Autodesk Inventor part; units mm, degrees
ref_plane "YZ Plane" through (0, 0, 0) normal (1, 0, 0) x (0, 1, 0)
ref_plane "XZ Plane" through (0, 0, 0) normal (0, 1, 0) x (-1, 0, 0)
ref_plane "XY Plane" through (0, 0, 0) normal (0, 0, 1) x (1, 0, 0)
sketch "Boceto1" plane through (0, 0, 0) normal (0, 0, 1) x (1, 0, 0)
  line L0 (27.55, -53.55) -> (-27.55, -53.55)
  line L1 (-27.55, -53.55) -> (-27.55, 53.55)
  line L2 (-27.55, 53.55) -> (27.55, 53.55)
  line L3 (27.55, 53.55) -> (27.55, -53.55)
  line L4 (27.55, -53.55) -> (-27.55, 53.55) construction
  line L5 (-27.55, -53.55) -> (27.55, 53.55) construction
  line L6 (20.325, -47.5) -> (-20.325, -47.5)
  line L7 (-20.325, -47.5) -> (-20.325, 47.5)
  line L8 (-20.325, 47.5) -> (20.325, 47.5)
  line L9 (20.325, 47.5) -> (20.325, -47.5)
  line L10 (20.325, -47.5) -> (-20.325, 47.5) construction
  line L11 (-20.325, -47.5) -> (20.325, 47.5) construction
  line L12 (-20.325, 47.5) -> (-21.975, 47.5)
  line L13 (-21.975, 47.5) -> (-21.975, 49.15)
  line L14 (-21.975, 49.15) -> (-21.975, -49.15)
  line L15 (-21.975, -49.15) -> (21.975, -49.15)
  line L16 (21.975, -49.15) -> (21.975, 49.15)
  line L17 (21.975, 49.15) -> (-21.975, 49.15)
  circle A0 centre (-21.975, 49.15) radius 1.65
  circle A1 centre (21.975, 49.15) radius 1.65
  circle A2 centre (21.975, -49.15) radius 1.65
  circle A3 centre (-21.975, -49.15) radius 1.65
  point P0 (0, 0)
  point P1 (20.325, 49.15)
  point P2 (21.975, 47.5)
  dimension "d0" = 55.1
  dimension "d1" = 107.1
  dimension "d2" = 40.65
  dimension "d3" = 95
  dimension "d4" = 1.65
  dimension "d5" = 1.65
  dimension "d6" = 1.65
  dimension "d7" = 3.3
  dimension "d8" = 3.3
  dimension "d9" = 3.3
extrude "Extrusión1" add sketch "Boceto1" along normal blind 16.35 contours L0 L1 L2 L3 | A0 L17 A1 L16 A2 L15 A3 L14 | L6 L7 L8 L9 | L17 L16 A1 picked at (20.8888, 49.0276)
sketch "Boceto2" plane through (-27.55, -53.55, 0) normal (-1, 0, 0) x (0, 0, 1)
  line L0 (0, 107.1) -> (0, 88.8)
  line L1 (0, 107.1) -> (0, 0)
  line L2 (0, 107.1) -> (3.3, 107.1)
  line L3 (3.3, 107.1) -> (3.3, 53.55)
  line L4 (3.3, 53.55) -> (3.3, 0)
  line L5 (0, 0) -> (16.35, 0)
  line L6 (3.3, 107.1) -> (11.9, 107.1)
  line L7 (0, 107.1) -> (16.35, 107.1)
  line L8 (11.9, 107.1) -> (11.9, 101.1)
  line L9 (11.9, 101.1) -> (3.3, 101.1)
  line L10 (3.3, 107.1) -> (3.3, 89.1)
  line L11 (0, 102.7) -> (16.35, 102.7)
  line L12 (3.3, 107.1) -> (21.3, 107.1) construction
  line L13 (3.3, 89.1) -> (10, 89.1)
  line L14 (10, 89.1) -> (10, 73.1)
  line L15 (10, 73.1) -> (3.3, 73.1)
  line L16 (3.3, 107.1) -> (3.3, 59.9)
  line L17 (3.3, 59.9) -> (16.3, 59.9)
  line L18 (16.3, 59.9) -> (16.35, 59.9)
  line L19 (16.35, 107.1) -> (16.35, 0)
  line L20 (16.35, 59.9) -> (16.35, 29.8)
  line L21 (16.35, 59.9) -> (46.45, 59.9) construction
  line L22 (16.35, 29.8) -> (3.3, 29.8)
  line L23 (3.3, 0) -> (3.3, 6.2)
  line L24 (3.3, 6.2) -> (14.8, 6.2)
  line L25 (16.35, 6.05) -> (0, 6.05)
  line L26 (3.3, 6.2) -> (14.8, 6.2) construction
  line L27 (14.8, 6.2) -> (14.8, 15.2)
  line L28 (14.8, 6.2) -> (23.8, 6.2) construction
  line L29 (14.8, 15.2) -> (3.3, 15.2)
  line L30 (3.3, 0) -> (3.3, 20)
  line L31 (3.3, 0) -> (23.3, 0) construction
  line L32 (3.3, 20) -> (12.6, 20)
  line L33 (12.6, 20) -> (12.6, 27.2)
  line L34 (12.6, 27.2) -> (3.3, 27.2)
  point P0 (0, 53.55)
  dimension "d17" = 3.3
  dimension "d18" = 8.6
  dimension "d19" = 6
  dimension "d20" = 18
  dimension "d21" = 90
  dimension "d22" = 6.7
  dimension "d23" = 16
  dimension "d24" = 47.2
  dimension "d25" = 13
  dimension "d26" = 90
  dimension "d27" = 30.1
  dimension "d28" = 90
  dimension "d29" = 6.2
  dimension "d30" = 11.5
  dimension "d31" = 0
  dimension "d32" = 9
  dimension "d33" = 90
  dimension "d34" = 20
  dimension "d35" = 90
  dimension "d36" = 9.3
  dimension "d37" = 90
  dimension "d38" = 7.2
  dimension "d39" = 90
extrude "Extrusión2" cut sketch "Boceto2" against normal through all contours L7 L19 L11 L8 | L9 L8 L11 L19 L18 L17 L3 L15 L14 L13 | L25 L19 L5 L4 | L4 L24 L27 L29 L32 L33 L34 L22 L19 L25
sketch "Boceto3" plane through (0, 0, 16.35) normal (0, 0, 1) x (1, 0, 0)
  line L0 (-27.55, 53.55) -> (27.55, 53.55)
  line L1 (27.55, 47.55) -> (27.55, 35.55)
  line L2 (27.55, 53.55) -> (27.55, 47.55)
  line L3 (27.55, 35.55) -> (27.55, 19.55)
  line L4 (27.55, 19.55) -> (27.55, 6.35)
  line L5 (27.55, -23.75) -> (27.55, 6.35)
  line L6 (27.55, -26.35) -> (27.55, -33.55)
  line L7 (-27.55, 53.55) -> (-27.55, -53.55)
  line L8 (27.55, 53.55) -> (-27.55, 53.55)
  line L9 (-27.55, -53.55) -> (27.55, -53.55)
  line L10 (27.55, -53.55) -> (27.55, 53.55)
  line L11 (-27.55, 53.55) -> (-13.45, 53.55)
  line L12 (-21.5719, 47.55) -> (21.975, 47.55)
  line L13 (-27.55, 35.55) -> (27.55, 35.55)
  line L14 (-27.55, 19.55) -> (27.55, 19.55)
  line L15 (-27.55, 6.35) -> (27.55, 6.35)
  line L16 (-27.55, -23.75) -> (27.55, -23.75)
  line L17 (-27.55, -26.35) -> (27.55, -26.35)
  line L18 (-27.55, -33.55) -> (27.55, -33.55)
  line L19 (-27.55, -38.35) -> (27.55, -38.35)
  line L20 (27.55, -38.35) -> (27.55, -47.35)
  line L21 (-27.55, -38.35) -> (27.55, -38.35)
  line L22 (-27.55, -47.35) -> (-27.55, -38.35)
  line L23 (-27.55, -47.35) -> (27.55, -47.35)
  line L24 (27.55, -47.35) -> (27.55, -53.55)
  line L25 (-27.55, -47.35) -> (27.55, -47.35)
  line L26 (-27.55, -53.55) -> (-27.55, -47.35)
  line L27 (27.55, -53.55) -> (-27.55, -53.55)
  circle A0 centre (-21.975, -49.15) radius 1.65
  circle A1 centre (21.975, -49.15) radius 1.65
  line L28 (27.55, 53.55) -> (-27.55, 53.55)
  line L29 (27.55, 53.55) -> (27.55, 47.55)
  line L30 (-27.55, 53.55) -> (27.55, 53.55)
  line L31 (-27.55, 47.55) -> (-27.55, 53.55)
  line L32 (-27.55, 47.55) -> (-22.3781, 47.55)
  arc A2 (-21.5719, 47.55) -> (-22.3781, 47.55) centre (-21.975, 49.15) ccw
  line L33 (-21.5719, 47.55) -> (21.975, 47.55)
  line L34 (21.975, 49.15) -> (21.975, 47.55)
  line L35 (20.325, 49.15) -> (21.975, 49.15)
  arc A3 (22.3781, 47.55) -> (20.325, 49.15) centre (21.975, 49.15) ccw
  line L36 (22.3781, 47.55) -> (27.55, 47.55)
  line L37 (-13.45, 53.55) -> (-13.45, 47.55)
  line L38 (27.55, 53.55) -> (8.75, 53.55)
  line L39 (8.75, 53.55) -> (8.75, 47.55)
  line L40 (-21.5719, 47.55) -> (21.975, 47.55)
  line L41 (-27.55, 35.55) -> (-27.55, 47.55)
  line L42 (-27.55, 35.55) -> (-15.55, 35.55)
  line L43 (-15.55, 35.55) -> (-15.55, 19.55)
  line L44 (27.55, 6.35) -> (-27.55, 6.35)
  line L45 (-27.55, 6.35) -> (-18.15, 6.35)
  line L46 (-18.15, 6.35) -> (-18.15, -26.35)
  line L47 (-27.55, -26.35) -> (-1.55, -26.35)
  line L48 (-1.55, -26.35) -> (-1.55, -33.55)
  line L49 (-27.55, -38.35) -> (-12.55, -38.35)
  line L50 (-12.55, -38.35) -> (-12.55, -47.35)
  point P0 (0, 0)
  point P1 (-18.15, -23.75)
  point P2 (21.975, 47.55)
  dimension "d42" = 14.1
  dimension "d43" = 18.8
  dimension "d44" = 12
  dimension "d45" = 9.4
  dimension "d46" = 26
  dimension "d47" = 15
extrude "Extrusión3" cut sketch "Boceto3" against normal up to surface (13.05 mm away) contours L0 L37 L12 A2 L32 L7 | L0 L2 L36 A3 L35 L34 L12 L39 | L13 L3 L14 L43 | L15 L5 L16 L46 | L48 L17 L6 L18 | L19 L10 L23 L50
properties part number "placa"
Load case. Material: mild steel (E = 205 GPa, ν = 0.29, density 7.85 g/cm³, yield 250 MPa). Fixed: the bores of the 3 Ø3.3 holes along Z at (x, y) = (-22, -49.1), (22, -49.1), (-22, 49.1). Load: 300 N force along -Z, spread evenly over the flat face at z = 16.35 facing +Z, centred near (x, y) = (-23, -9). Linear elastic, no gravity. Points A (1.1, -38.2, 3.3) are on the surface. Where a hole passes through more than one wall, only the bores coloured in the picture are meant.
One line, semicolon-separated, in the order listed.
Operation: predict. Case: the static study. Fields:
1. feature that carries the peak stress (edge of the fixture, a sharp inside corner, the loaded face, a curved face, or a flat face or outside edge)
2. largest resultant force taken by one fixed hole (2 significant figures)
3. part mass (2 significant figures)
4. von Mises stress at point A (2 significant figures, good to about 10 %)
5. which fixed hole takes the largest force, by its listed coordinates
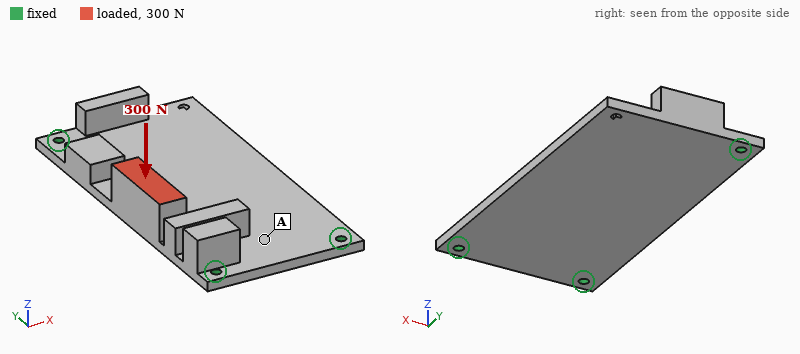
edge of the fixture; 200 N; 230 g; 9.3 MPa; (-22, -49.1)
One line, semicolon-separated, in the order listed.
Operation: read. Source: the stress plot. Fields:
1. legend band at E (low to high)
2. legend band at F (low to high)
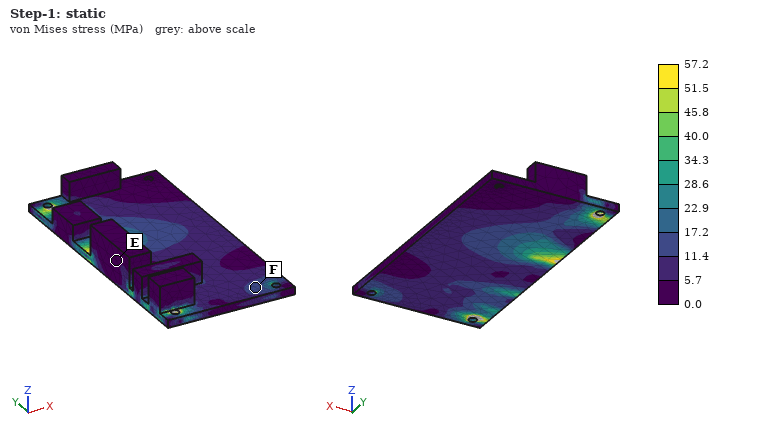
0.0 to 5.7 MPa; 11.4 to 17.2 MPa
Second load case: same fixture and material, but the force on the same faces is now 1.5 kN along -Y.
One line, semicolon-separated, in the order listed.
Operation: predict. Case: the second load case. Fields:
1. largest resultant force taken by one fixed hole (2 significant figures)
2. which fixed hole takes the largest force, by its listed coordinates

820 N; (-22, -49.1)
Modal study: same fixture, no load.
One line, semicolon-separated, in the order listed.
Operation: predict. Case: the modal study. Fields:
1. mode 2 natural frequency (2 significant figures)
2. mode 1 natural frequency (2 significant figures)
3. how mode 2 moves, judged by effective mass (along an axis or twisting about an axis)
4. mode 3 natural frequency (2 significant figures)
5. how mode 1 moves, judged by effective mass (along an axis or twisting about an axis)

1700 Hz; 1100 Hz; along Z; 2800 Hz; along Z
